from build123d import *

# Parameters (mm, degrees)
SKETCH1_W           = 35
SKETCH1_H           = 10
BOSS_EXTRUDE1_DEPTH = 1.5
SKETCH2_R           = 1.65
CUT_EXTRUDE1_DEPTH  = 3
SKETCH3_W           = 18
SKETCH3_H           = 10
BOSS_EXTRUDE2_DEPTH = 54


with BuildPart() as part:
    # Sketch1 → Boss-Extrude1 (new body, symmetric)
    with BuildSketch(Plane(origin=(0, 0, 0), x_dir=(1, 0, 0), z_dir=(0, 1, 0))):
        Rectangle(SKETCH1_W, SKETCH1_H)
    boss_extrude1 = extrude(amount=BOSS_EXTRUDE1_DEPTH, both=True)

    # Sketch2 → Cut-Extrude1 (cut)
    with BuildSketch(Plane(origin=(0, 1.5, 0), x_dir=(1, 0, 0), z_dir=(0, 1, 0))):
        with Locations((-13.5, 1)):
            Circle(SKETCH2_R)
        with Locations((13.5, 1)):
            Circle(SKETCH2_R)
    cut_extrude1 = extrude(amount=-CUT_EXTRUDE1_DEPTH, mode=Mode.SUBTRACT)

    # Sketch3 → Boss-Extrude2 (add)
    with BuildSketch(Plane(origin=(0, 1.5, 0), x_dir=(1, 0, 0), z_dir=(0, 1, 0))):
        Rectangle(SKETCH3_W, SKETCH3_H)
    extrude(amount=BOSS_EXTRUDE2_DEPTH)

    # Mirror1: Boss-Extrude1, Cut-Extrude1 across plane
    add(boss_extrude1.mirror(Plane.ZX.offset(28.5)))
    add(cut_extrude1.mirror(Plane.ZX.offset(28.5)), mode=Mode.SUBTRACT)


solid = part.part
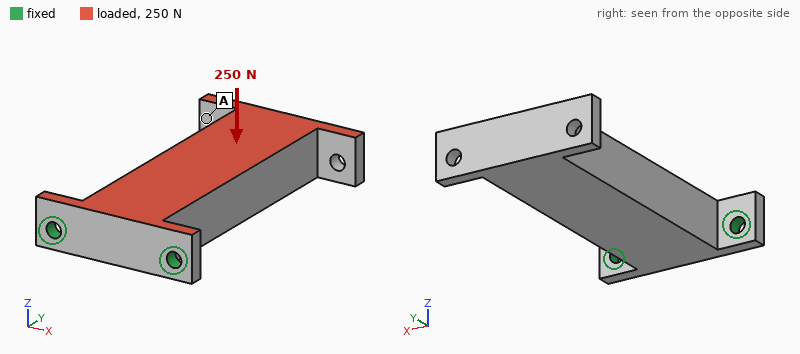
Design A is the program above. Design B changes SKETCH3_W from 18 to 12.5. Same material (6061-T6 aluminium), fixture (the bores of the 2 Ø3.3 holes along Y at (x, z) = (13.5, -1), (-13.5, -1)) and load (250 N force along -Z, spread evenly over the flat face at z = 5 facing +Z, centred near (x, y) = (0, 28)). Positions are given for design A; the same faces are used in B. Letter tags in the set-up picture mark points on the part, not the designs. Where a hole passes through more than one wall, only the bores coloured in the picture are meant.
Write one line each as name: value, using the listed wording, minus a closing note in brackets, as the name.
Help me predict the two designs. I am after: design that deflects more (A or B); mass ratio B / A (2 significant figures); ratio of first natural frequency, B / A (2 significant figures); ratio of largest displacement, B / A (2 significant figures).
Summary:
design that deflects more: B
mass ratio B / A: 0.75
ratio of first natural frequency, B / A: 0.90
ratio of largest displacement, B / A: 1.6
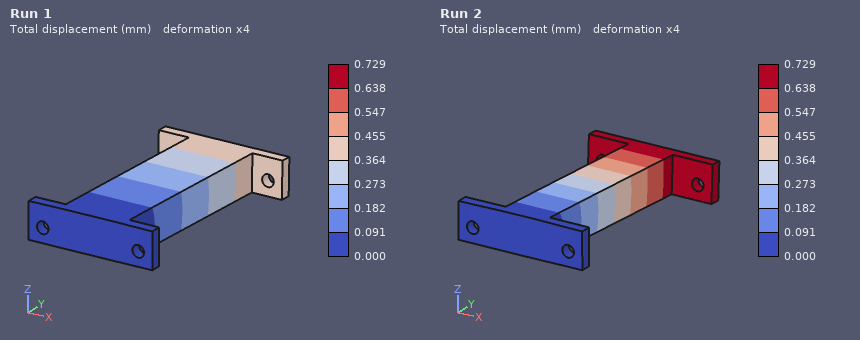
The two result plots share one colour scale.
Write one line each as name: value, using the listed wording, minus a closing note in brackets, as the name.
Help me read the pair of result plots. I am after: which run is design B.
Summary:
which run is design B: Run 2
